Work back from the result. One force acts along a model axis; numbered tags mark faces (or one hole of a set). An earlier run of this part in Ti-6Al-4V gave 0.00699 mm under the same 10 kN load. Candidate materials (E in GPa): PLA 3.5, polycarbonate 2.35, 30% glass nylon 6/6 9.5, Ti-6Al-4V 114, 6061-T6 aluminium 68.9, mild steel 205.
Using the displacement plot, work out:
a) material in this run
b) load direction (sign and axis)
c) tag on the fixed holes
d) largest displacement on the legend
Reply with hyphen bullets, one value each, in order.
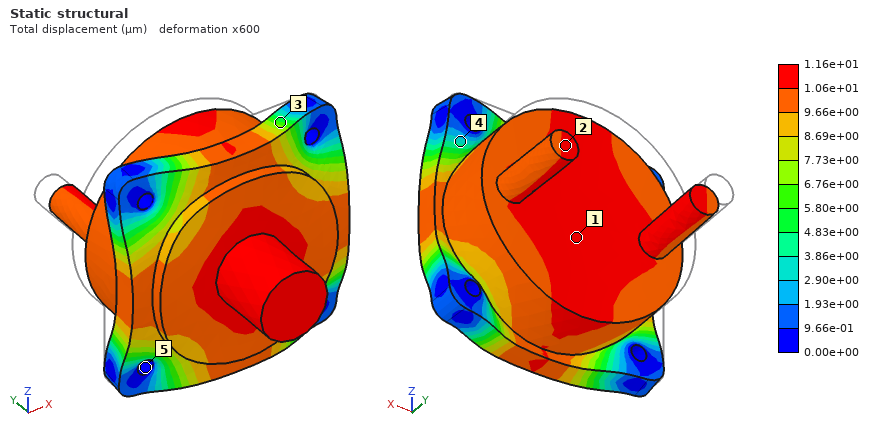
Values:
- 6061-T6 aluminium
- -Y
- 5
- 1.16e+01 µm
